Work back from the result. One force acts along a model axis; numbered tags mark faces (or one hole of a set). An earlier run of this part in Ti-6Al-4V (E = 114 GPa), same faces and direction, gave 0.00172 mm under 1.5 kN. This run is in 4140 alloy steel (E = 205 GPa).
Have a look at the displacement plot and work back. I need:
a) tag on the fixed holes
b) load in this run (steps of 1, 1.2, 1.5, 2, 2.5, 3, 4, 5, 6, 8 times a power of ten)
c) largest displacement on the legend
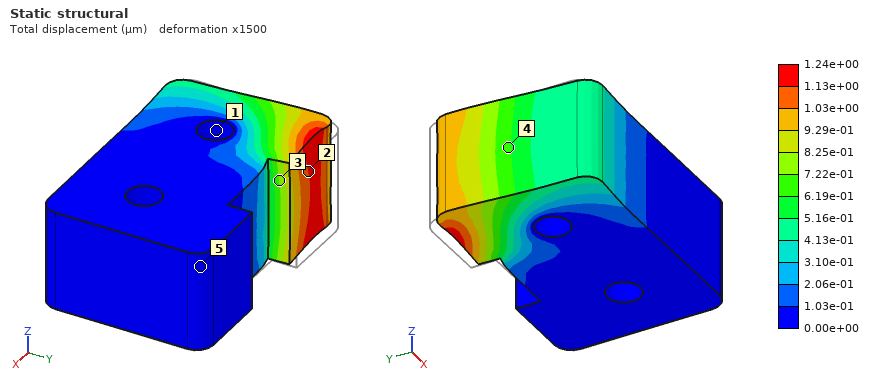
1
2 kN
1.24e+00 µm
